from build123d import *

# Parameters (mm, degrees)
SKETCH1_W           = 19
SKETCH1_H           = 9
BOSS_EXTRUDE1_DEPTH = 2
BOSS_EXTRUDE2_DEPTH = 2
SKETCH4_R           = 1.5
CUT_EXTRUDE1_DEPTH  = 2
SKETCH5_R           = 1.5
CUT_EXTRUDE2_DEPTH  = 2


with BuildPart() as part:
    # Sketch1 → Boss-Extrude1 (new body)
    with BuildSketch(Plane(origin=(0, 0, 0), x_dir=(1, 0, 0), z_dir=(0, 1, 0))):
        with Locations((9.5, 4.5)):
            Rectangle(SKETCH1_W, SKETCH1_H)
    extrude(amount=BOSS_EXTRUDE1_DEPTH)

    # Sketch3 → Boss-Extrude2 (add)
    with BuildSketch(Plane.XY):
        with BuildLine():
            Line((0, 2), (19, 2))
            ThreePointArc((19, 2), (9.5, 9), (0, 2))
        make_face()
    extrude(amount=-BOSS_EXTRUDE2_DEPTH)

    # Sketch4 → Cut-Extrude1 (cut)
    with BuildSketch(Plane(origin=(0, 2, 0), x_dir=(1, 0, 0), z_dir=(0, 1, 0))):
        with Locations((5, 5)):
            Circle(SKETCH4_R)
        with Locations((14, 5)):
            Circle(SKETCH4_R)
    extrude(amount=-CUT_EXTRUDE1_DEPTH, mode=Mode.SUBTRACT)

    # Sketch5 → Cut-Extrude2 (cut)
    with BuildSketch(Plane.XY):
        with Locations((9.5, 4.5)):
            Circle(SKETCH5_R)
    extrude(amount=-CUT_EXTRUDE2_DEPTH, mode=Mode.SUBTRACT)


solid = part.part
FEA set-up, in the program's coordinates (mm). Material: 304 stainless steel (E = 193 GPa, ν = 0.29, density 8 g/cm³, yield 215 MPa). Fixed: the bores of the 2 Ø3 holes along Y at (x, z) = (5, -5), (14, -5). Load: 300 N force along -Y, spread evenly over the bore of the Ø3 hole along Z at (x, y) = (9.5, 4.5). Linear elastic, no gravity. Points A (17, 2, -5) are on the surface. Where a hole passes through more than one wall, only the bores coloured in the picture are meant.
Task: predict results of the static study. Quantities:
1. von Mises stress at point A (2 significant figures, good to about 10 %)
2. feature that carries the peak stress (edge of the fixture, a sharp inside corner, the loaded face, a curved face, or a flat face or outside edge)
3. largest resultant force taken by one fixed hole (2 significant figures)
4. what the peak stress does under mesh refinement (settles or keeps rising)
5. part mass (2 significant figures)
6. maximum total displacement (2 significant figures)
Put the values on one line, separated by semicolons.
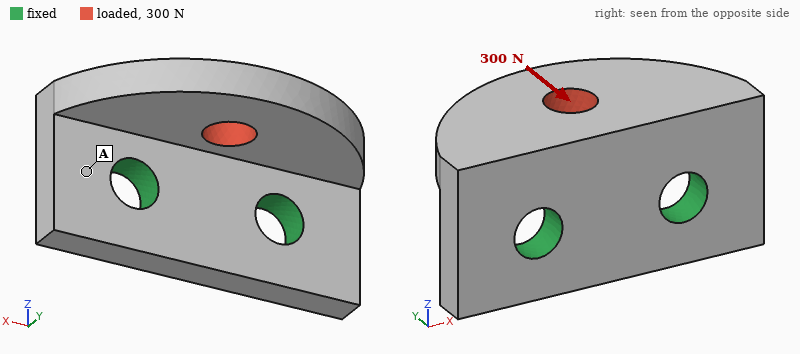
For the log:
17 MPa; edge of the fixture; 150 N; keeps rising; 4.0 g; 6.7 µm
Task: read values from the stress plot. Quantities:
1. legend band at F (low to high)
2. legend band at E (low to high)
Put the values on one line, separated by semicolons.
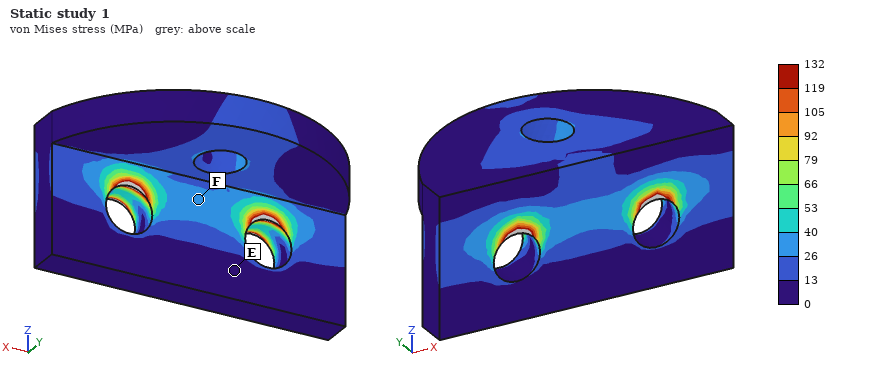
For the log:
26 to 40 MPa; 0 to 13 MPa
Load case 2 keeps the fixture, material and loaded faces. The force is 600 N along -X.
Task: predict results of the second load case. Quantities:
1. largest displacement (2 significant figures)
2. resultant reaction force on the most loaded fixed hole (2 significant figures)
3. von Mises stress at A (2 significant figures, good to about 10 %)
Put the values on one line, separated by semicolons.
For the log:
5.2 µm; 390 N; 29 MPa
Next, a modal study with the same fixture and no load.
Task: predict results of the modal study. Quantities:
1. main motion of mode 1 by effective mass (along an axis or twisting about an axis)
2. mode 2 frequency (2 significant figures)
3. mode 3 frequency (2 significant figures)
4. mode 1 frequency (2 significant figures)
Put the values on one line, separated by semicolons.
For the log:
along Z; 34 kHz; 53 kHz; 20 kHz
